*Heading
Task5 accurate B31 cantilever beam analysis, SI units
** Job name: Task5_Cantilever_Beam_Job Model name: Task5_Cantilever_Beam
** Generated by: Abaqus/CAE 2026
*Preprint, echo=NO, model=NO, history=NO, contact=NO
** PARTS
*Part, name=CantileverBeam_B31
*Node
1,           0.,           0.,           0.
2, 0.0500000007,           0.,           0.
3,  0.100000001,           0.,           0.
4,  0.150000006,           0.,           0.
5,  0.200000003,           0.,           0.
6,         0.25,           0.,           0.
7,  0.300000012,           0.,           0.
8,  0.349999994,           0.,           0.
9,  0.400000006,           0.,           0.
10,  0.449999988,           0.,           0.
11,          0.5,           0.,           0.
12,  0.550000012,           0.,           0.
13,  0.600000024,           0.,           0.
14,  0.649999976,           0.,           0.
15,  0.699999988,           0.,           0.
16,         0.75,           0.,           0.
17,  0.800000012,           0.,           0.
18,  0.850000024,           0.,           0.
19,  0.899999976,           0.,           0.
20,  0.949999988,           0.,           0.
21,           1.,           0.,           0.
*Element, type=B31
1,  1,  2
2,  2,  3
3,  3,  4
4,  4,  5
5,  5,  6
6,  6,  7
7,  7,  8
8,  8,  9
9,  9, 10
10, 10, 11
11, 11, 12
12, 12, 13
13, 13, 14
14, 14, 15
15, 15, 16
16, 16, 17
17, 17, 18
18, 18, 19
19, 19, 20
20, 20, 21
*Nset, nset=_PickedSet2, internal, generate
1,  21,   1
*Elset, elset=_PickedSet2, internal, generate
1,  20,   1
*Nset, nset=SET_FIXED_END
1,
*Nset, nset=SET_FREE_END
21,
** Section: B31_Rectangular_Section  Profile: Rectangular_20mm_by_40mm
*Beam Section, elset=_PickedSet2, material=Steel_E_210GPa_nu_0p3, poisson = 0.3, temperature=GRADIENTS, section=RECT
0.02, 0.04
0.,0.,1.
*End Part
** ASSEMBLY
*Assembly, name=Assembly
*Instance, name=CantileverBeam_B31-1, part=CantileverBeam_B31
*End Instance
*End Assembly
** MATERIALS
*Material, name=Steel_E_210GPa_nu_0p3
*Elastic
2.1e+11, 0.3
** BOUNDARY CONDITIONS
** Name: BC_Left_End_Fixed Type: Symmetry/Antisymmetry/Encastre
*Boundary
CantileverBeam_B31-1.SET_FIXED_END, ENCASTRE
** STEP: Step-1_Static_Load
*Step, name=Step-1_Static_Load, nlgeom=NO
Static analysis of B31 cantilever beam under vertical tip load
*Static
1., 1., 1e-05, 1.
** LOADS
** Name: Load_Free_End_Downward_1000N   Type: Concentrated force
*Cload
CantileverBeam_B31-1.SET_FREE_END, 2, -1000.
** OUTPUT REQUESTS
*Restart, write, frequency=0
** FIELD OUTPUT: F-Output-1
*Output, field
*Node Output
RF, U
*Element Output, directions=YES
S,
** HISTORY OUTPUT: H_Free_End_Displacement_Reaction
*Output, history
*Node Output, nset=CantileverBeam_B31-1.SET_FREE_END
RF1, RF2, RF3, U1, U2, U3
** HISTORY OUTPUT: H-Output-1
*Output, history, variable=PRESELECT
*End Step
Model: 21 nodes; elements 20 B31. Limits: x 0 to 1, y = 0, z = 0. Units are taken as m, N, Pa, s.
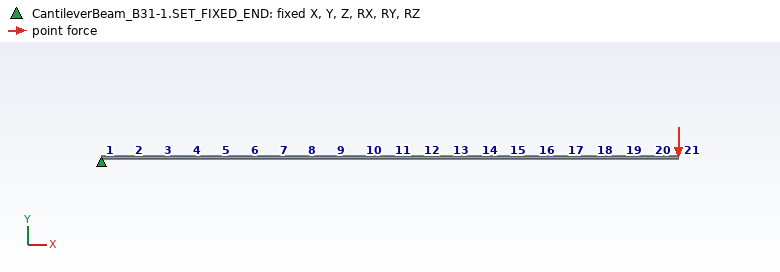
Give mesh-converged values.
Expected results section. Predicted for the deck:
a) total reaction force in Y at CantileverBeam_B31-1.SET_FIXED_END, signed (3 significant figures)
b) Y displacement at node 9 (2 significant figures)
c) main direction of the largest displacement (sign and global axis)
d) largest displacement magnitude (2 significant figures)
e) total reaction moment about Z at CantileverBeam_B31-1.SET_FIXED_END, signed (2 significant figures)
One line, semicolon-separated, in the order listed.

1000 N; -0.0031 m; -Y; 0.015 m; 1000 N·m
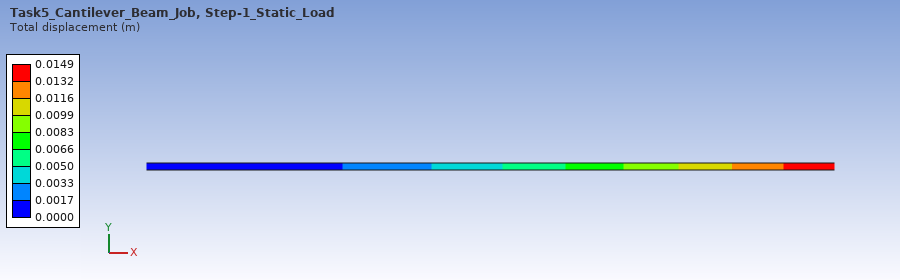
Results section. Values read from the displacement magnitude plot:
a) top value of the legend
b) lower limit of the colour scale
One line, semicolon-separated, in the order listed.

0.0149 m; 0.0000 m
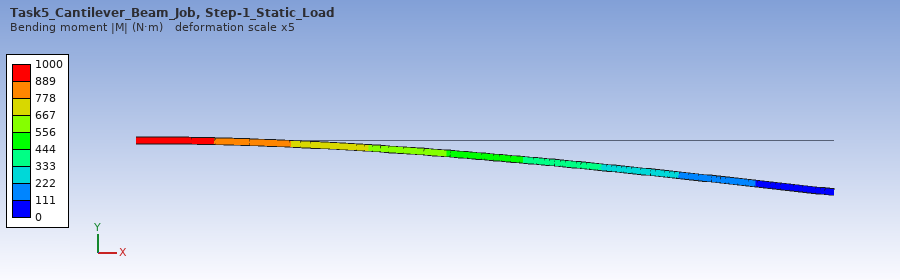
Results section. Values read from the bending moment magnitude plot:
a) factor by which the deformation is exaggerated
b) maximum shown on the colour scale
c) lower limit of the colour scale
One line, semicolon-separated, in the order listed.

5; 1000 N·m; 0 N·m
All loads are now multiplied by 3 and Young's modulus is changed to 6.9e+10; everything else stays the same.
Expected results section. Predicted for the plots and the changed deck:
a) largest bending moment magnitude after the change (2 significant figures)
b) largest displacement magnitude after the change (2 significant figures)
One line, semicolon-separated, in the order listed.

3000 N·m; 0.14 m
